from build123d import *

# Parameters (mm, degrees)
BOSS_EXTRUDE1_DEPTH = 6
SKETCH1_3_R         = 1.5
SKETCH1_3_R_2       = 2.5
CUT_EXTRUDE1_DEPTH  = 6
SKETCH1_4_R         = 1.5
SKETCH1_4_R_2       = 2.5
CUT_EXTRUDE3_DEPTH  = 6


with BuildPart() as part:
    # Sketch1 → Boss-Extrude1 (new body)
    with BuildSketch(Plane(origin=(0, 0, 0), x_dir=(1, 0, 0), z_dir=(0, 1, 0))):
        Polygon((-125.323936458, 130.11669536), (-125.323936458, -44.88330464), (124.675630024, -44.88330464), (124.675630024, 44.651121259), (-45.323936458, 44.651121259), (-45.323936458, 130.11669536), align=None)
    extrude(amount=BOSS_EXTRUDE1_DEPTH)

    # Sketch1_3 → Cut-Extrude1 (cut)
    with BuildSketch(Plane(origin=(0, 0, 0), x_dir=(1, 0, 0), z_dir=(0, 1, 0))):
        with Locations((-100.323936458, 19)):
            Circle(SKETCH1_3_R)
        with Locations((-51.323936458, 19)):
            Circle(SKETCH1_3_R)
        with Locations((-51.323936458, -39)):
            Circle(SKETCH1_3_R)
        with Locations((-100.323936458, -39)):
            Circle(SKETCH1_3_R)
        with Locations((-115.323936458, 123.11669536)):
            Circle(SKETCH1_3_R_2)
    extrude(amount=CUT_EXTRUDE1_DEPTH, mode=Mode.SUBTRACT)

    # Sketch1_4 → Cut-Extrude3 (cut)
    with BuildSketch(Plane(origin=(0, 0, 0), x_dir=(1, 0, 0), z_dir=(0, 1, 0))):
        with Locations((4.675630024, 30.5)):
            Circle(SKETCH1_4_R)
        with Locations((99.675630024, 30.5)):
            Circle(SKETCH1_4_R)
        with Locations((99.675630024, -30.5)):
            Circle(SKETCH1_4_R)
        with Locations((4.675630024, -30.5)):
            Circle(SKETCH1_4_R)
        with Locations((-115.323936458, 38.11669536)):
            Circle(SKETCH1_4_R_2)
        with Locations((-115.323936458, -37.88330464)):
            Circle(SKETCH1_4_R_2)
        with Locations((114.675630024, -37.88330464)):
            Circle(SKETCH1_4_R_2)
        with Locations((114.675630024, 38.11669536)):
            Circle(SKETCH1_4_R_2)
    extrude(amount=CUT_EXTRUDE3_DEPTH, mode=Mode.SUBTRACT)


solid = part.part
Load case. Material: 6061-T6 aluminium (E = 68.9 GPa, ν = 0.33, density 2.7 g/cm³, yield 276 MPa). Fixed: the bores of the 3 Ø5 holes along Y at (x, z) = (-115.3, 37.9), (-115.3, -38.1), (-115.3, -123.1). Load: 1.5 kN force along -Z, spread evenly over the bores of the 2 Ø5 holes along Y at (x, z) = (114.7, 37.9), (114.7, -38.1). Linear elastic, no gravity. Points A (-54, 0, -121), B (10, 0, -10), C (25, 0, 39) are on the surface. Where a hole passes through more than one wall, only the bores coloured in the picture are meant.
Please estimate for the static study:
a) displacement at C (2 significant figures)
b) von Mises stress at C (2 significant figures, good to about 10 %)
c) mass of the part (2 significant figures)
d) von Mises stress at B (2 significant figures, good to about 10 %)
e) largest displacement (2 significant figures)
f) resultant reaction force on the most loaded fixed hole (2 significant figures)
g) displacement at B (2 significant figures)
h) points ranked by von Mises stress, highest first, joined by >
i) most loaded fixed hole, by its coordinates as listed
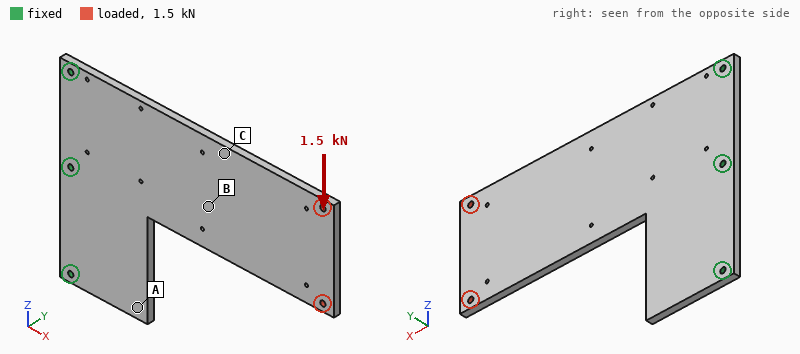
0.096 mm
15 MPa
470 g
8.4 MPa
0.23 mm
3.0 kN
0.066 mm
C > B > A
(-115.3, 37.9)
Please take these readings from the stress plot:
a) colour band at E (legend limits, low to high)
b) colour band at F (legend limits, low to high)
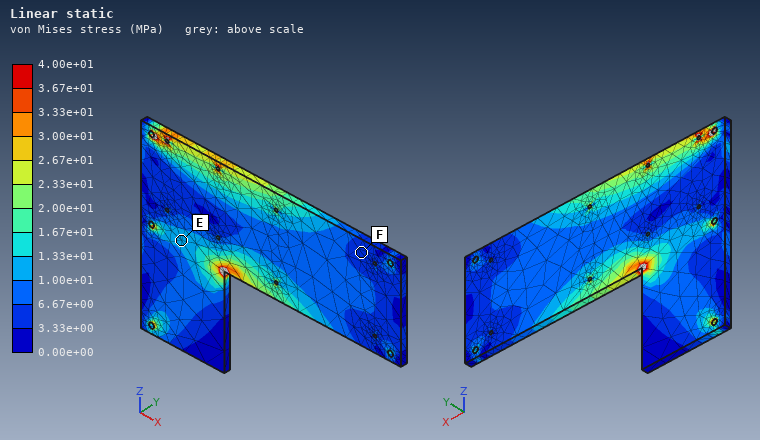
1.00e+01 to 1.33e+01 MPa
3.33e+00 to 6.67e+00 MPa
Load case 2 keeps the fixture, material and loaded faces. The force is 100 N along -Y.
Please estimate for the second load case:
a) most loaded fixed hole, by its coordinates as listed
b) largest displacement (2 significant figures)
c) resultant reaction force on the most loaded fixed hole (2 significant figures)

(-115.3, -38.1)
3.5 mm
110 N
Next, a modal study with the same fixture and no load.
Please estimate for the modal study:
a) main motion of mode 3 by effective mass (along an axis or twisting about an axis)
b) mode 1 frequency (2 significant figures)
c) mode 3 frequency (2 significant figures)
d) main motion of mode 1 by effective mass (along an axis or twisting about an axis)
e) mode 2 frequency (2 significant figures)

along Y
91 Hz
530 Hz
along Y
490 Hz
